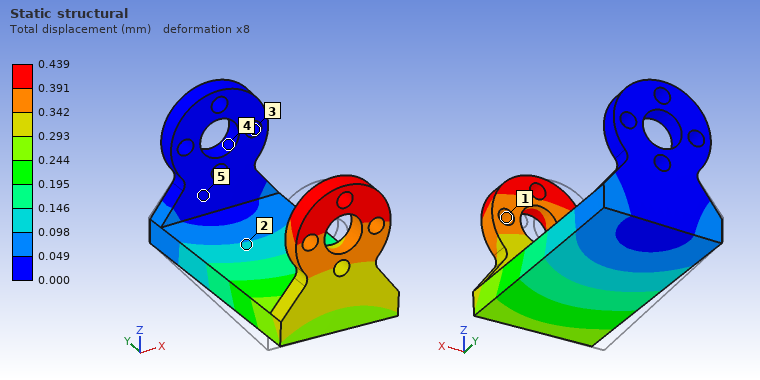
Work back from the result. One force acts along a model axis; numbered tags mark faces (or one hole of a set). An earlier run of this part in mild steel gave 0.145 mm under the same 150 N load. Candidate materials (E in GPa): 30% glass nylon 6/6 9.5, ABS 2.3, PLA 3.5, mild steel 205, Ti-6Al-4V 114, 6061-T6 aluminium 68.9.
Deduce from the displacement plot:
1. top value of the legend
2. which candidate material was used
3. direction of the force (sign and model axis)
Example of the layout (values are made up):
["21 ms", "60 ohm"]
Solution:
["0.439 mm", "6061-T6 aluminium", "+X"]
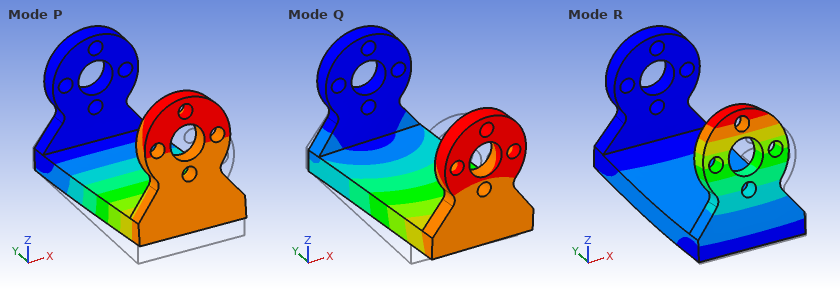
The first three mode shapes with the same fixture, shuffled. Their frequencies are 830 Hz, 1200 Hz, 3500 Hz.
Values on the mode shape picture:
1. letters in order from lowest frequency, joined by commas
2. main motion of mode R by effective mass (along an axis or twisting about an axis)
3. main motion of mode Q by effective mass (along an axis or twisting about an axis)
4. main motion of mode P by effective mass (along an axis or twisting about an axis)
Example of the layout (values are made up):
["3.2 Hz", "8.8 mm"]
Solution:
["P, Q, R", "along Y", "along X", "along Z"]
